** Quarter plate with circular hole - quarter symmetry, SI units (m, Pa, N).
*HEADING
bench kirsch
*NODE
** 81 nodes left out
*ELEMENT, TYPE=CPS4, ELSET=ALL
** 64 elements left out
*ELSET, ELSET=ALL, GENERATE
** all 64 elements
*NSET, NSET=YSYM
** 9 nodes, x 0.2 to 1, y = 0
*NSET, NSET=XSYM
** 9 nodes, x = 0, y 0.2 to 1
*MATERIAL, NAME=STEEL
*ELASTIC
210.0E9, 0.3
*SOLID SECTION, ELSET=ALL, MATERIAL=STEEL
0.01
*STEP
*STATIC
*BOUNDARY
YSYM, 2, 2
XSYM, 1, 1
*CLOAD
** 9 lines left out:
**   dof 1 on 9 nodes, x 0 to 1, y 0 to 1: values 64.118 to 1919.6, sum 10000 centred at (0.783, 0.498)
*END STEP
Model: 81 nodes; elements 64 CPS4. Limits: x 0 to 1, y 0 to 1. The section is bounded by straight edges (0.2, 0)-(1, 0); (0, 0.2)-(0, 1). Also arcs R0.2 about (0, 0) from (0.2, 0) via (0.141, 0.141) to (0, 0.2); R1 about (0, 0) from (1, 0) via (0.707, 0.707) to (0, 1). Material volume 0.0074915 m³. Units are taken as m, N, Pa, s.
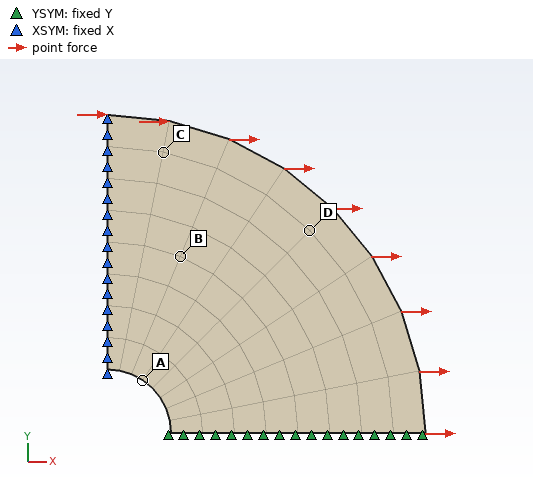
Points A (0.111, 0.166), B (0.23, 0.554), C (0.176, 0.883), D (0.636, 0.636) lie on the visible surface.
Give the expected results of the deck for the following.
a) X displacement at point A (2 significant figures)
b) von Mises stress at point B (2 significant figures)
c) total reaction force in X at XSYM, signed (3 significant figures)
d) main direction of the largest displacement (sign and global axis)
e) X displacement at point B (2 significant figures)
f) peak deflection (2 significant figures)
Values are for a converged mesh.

1.8e-06 m
1.2e+06 Pa
-10000 N
+X
1.2e-06 m
7.2e-06 m
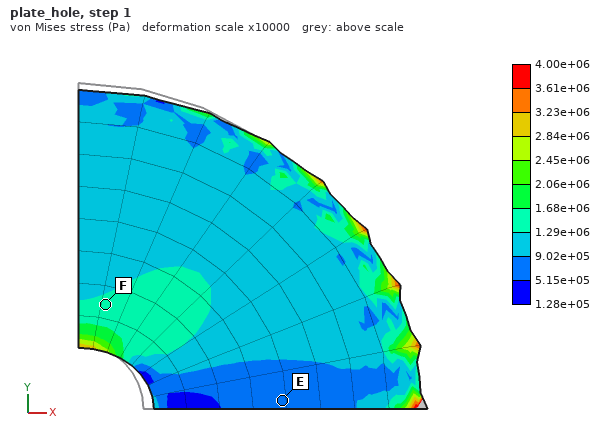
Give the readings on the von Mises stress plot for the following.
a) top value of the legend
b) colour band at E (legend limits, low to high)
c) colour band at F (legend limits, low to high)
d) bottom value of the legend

4.00e+06 Pa
5.15e+05 to 9.02e+05 Pa
1.29e+06 to 1.68e+06 Pa
1.28e+05 Pa
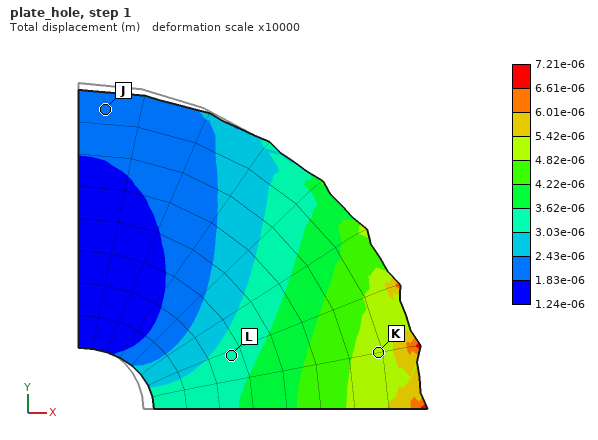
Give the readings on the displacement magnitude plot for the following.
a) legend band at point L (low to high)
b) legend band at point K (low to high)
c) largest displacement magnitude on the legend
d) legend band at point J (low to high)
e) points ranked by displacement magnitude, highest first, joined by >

3.03e-06 to 3.62e-06 m
4.82e-06 to 5.42e-06 m
7.21e-06 m
1.83e-06 to 2.43e-06 m
K > L > J
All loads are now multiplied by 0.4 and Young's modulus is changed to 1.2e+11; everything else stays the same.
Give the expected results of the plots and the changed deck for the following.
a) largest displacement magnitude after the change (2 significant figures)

5.0e-06 m
